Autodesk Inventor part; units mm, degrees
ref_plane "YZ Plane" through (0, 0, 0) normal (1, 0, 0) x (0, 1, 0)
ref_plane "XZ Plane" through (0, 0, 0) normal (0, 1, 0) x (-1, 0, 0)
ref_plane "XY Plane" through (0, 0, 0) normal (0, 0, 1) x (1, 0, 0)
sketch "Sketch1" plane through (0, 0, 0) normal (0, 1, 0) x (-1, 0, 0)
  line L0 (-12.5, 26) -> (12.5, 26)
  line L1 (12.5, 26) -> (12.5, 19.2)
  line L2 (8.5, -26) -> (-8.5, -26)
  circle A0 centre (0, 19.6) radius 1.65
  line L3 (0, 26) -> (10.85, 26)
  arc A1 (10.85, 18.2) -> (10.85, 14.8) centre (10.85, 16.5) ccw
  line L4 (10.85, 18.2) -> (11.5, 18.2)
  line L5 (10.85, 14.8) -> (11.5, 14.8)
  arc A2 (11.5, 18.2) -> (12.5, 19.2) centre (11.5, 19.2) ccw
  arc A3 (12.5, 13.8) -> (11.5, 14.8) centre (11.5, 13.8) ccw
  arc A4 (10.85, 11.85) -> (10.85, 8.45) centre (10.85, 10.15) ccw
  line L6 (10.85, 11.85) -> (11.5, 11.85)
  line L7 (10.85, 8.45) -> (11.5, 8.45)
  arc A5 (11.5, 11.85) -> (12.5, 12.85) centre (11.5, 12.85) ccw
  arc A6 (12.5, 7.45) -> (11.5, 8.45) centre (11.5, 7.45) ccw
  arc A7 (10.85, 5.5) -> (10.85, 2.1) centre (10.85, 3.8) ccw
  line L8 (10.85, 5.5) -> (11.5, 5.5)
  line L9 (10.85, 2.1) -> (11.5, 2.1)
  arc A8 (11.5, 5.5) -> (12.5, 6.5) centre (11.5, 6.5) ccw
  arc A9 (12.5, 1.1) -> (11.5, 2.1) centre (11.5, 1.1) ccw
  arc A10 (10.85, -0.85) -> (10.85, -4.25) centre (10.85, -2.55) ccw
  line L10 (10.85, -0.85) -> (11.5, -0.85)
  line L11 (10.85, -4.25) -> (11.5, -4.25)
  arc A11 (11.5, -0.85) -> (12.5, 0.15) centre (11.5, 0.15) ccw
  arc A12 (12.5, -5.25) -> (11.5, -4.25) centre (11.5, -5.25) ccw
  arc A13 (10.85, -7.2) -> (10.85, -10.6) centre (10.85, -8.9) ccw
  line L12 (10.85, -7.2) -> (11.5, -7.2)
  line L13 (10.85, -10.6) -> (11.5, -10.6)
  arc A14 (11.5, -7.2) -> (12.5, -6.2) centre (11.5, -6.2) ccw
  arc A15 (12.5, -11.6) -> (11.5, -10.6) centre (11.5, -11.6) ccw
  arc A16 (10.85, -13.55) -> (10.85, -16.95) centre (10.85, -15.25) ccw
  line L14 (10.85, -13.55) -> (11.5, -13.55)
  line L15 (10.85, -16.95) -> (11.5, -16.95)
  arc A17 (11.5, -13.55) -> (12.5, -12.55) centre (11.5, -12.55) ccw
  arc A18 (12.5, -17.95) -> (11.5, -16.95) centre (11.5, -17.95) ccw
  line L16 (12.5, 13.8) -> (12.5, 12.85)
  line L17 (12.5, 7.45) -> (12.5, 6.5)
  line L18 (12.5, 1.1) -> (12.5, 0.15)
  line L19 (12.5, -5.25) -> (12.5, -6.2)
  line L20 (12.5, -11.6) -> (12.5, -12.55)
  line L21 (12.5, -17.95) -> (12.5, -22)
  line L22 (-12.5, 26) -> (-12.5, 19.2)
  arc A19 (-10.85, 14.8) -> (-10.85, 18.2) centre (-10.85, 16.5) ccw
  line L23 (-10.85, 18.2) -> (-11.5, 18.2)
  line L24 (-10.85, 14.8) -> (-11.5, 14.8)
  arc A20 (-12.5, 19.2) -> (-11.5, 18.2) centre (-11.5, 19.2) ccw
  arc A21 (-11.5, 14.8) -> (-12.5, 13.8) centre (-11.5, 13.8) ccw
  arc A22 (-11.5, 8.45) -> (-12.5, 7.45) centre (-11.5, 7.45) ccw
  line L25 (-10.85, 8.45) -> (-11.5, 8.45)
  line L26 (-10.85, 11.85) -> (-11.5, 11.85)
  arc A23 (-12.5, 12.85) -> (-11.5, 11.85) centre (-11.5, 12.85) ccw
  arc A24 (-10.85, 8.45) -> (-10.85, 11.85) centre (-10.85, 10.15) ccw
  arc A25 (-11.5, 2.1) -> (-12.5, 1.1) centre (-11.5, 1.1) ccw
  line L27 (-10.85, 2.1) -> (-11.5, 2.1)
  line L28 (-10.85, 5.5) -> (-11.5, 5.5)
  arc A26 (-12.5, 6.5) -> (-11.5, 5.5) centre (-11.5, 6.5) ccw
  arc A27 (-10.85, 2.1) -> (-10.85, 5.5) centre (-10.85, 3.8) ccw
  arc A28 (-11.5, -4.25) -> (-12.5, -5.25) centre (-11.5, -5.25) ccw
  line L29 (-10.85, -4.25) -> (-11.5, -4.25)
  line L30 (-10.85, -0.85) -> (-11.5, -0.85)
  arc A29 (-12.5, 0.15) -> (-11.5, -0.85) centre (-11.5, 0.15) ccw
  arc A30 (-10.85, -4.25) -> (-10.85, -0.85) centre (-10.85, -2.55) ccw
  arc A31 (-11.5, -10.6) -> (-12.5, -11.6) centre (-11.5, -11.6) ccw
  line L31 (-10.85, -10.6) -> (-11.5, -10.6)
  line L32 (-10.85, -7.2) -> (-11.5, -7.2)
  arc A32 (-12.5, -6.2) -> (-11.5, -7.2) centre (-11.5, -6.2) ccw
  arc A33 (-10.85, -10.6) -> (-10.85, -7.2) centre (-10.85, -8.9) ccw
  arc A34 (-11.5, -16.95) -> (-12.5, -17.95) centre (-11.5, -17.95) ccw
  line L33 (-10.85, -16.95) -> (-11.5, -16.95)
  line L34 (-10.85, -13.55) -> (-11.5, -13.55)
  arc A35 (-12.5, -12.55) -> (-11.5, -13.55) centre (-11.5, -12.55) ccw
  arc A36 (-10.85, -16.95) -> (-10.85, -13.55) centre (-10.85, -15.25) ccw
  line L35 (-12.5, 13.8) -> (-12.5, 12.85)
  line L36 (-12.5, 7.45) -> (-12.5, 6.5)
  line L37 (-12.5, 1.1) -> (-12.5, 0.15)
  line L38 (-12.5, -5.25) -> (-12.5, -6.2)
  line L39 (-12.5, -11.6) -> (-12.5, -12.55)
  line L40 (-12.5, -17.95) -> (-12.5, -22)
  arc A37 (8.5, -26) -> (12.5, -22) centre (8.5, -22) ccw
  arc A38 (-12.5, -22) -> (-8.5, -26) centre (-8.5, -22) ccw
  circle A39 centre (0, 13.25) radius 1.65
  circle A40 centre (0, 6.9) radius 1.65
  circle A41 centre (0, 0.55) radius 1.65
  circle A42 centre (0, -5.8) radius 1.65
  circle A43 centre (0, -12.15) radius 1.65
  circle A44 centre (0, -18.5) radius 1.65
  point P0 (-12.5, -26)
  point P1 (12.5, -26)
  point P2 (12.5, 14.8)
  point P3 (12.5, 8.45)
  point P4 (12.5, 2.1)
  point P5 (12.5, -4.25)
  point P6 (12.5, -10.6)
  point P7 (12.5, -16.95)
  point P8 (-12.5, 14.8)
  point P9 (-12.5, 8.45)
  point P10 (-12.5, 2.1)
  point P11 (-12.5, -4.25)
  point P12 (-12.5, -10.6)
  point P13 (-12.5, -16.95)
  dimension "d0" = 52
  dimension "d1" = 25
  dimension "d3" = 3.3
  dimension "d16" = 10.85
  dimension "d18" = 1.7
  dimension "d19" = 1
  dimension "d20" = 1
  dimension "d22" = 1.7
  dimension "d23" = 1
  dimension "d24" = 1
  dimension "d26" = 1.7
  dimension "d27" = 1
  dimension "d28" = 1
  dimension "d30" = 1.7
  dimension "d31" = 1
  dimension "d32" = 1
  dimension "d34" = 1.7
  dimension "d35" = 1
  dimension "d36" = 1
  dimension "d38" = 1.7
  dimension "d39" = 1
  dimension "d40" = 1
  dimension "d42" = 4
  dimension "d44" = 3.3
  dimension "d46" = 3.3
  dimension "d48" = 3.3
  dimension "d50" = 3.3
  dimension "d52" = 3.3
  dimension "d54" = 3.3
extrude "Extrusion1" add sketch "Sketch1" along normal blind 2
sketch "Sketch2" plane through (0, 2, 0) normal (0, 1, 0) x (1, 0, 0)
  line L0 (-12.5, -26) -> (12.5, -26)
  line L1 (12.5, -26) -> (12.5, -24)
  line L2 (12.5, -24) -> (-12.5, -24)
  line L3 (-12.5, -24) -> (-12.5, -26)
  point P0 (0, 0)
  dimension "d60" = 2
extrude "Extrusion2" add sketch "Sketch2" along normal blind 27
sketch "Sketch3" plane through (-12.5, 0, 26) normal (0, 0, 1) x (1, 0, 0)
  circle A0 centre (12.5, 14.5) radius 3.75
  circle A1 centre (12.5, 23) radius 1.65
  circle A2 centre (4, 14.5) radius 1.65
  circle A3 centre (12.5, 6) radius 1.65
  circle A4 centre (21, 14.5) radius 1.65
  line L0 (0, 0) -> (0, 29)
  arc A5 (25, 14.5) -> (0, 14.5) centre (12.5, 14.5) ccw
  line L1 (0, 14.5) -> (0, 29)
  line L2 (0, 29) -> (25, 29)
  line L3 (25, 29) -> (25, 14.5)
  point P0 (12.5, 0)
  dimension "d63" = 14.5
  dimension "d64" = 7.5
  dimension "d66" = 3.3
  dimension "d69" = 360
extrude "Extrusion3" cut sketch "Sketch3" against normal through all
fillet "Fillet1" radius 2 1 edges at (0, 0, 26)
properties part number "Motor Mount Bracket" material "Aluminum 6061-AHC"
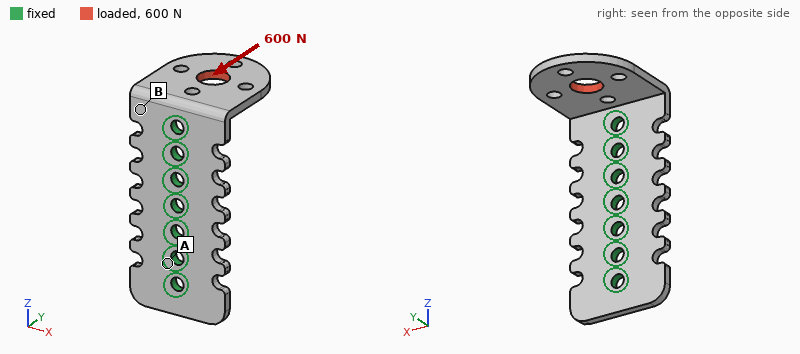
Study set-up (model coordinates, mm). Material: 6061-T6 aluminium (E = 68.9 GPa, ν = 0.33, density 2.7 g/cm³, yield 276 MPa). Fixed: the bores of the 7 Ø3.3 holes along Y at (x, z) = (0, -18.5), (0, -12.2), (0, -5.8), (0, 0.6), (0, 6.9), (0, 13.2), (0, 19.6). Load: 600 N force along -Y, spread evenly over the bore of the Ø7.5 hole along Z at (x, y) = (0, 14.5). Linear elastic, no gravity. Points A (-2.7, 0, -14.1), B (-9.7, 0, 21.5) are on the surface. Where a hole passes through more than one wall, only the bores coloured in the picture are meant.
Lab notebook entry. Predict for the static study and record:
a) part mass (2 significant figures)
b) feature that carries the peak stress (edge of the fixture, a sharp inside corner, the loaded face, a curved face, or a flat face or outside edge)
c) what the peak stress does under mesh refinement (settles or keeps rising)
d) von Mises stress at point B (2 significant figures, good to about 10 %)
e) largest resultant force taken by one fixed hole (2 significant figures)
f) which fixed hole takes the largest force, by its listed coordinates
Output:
8.5 g
edge of the fixture
keeps rising
40 MPa
710 N
(0, 19.6)
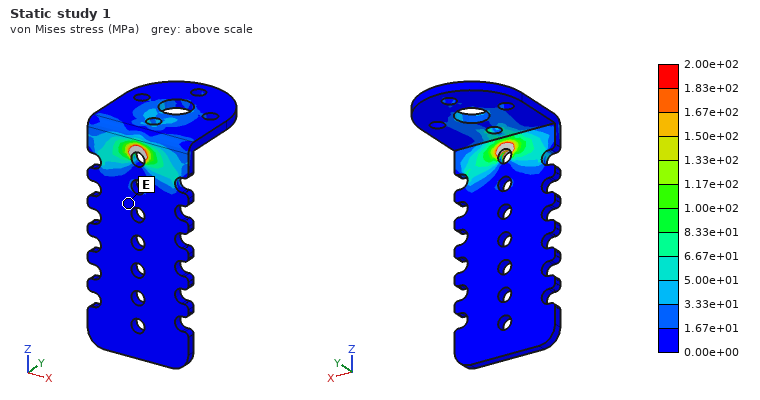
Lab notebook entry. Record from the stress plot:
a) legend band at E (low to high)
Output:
0.00e+00 to 1.67e+01 MPa
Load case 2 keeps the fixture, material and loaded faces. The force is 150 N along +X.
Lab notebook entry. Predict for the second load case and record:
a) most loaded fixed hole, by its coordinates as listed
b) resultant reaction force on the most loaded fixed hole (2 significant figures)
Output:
(0, 19.6)
170 N
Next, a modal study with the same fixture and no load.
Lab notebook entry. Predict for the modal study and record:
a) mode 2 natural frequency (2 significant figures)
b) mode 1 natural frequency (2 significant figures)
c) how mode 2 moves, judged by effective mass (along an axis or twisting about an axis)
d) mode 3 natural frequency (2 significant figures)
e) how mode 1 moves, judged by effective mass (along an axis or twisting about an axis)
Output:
3600 Hz
2200 Hz
along X
6700 Hz
along Z
